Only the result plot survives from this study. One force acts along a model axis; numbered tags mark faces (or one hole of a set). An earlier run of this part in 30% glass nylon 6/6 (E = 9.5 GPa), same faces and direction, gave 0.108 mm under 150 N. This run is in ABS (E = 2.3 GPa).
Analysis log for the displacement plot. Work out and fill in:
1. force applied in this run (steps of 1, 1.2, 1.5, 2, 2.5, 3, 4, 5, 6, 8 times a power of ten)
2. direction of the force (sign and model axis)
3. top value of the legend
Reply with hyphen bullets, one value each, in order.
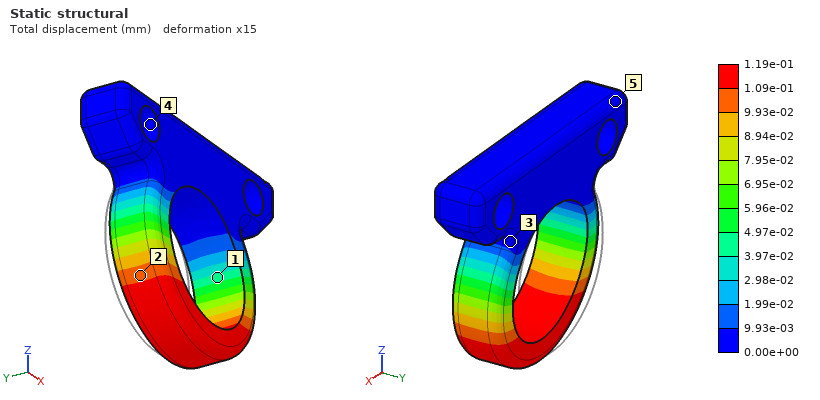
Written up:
- 40 N
- +X
- 1.19e-01 mm
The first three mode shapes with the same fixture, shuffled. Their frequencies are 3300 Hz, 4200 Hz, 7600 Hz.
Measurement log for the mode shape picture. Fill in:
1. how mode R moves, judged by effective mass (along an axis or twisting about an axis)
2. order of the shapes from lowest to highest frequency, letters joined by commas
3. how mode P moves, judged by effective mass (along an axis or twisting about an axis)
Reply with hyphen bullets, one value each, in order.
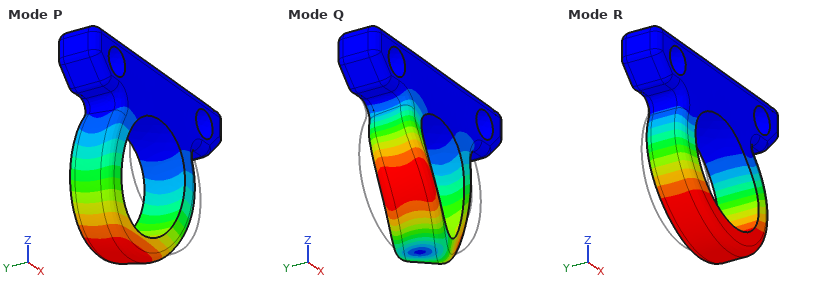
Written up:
- along X
- P, R, Q
- along Y
